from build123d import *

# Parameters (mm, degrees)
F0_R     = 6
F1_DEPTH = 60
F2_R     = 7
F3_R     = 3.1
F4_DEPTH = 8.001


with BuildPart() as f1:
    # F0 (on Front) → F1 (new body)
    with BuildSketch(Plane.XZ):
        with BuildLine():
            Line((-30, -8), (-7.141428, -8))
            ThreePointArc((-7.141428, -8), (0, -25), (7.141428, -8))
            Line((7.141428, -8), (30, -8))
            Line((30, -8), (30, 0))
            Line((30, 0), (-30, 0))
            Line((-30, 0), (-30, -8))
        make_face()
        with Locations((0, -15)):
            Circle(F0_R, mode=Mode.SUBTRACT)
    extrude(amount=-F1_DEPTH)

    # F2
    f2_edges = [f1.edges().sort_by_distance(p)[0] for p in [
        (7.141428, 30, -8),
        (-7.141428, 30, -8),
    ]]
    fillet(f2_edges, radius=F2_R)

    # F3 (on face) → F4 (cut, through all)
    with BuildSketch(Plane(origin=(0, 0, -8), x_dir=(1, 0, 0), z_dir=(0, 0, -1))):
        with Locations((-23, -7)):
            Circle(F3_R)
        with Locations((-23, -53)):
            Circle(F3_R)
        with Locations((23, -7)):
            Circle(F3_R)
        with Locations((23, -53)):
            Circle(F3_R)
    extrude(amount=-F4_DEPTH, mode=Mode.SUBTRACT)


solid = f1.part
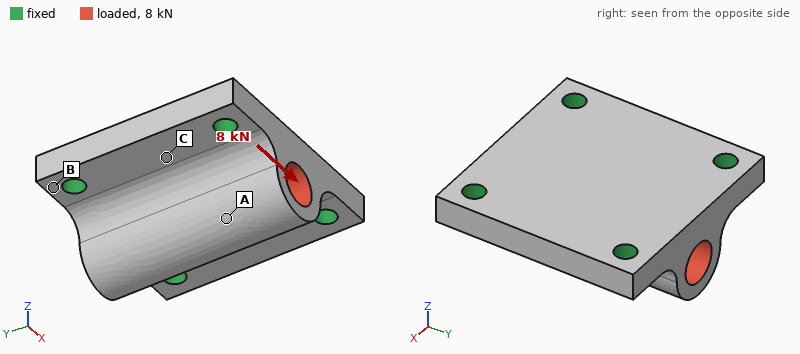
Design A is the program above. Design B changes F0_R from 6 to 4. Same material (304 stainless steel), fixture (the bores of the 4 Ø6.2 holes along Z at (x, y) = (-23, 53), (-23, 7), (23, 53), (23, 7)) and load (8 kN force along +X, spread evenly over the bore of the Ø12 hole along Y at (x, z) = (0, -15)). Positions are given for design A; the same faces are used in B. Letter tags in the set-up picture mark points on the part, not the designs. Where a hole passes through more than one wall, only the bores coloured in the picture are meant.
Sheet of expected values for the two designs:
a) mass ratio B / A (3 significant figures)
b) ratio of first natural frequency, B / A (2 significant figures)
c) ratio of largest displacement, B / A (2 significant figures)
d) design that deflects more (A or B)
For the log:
1.09
1.00
0.72
A
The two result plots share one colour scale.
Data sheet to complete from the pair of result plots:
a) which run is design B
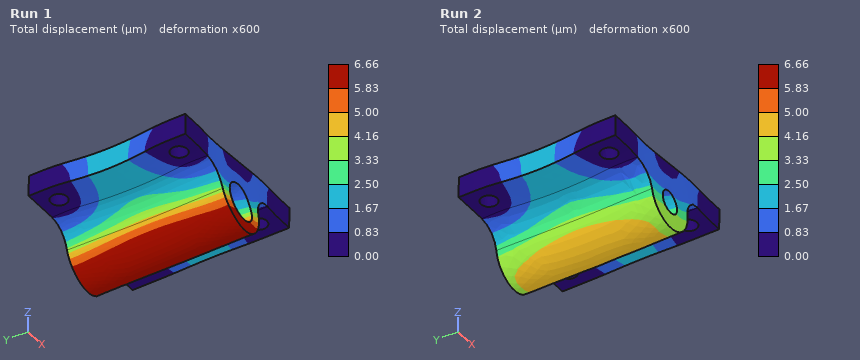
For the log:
Run 2
